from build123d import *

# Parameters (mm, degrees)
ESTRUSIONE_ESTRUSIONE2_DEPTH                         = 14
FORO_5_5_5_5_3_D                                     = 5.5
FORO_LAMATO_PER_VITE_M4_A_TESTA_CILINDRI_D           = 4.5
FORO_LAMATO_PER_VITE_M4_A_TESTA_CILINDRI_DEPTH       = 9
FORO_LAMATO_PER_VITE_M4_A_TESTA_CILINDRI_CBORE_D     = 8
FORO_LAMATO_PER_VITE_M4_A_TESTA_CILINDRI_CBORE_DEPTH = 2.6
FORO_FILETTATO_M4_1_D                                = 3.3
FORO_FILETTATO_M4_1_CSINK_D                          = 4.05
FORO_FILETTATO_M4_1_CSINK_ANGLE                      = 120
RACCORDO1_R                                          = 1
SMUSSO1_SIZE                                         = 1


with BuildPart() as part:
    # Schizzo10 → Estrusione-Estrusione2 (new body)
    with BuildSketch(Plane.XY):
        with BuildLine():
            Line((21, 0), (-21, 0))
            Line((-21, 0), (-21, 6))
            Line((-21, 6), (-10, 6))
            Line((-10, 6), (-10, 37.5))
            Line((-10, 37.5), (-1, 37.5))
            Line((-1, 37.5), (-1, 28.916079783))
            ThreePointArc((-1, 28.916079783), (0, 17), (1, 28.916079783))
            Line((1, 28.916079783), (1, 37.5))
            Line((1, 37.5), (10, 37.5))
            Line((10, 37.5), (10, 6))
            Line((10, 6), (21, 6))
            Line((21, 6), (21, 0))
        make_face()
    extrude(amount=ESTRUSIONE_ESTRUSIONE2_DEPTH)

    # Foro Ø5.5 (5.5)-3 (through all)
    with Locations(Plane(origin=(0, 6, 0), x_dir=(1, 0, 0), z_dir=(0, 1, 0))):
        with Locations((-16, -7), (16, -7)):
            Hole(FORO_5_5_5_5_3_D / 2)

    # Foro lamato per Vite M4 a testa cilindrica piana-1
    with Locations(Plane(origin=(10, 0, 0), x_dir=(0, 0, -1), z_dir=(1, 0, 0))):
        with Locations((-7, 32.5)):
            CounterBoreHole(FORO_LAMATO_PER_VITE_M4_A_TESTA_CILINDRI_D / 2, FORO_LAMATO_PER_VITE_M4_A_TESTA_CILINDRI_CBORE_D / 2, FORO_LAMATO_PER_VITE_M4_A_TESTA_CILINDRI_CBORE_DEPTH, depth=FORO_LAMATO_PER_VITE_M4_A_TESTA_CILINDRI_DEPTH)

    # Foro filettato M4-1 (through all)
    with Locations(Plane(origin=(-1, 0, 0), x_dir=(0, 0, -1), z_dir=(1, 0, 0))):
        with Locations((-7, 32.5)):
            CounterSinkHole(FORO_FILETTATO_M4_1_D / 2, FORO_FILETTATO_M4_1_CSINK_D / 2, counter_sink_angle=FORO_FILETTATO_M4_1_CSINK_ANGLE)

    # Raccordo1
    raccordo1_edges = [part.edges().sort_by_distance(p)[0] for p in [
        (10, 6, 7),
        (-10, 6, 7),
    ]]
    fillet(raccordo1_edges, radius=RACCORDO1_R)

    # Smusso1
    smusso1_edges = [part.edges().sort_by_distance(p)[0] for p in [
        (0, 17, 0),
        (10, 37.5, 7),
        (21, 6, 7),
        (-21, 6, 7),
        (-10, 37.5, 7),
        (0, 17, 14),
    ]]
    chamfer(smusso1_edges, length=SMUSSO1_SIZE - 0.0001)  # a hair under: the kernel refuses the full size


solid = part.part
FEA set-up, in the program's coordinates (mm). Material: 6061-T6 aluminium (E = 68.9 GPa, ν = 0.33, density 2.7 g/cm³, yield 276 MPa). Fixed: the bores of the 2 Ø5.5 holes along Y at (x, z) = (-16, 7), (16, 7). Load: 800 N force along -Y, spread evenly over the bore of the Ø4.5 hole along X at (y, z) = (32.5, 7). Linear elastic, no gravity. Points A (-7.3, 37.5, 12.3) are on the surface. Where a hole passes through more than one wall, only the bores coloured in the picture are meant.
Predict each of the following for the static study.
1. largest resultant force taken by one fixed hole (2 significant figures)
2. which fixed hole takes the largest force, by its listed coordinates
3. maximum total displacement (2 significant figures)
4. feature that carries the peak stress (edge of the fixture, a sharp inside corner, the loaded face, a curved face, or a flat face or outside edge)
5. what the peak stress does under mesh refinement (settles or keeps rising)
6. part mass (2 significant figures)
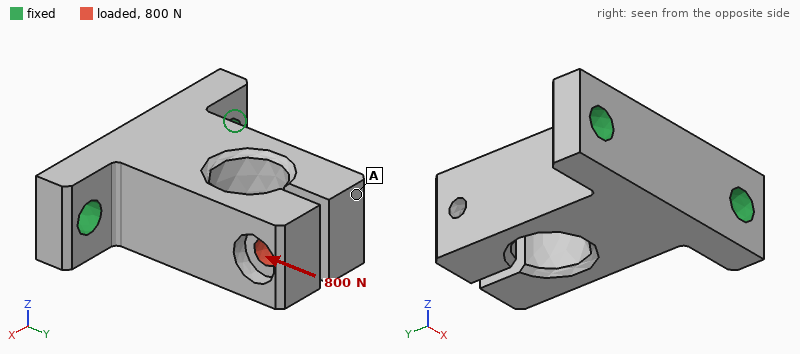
560 N
(16, 7)
77 µm
a sharp inside corner
keeps rising
27 g
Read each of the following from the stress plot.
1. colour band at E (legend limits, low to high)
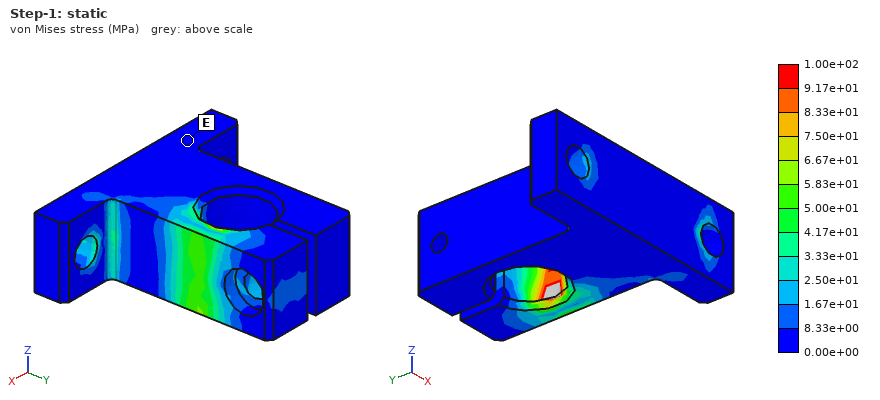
0.00e+00 to 8.33e+00 MPa
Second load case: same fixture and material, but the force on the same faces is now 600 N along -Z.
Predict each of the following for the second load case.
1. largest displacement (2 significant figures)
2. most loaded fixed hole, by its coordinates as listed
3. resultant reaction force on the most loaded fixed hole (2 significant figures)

0.15 mm
(16, 7)
370 N
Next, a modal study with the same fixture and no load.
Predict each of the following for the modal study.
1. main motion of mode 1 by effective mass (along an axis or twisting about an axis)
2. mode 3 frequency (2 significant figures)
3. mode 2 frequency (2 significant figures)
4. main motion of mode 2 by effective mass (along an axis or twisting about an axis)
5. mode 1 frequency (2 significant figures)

along Z
6100 Hz
5500 Hz
along X
4500 Hz
